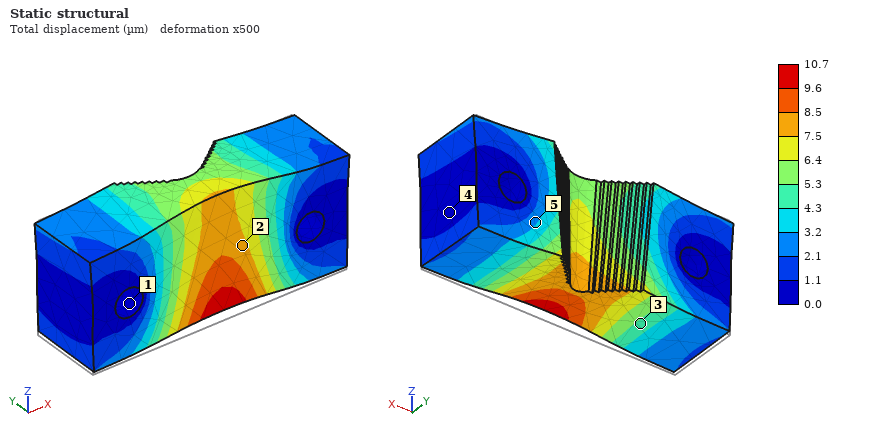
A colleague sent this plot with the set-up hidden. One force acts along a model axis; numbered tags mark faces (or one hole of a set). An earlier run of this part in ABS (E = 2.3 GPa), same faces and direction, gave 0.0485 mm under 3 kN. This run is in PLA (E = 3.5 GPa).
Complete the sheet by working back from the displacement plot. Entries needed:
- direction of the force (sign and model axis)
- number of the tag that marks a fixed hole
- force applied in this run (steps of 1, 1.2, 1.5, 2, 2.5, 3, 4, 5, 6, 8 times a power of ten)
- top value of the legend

+Z
1
1 kN
10.7 µm
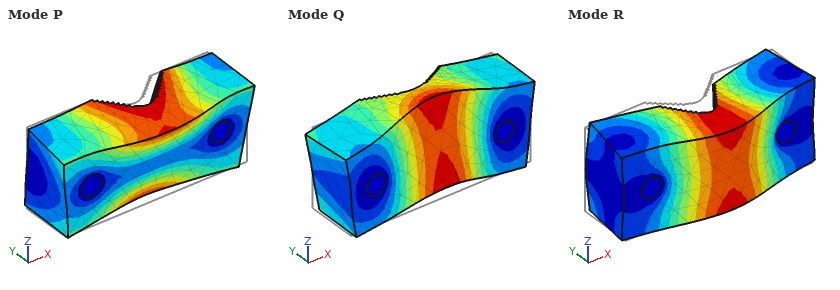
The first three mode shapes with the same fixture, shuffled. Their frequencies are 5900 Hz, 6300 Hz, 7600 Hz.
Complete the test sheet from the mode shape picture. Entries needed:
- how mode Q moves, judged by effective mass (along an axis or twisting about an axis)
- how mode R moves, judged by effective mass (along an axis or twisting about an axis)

along Z
along Y
